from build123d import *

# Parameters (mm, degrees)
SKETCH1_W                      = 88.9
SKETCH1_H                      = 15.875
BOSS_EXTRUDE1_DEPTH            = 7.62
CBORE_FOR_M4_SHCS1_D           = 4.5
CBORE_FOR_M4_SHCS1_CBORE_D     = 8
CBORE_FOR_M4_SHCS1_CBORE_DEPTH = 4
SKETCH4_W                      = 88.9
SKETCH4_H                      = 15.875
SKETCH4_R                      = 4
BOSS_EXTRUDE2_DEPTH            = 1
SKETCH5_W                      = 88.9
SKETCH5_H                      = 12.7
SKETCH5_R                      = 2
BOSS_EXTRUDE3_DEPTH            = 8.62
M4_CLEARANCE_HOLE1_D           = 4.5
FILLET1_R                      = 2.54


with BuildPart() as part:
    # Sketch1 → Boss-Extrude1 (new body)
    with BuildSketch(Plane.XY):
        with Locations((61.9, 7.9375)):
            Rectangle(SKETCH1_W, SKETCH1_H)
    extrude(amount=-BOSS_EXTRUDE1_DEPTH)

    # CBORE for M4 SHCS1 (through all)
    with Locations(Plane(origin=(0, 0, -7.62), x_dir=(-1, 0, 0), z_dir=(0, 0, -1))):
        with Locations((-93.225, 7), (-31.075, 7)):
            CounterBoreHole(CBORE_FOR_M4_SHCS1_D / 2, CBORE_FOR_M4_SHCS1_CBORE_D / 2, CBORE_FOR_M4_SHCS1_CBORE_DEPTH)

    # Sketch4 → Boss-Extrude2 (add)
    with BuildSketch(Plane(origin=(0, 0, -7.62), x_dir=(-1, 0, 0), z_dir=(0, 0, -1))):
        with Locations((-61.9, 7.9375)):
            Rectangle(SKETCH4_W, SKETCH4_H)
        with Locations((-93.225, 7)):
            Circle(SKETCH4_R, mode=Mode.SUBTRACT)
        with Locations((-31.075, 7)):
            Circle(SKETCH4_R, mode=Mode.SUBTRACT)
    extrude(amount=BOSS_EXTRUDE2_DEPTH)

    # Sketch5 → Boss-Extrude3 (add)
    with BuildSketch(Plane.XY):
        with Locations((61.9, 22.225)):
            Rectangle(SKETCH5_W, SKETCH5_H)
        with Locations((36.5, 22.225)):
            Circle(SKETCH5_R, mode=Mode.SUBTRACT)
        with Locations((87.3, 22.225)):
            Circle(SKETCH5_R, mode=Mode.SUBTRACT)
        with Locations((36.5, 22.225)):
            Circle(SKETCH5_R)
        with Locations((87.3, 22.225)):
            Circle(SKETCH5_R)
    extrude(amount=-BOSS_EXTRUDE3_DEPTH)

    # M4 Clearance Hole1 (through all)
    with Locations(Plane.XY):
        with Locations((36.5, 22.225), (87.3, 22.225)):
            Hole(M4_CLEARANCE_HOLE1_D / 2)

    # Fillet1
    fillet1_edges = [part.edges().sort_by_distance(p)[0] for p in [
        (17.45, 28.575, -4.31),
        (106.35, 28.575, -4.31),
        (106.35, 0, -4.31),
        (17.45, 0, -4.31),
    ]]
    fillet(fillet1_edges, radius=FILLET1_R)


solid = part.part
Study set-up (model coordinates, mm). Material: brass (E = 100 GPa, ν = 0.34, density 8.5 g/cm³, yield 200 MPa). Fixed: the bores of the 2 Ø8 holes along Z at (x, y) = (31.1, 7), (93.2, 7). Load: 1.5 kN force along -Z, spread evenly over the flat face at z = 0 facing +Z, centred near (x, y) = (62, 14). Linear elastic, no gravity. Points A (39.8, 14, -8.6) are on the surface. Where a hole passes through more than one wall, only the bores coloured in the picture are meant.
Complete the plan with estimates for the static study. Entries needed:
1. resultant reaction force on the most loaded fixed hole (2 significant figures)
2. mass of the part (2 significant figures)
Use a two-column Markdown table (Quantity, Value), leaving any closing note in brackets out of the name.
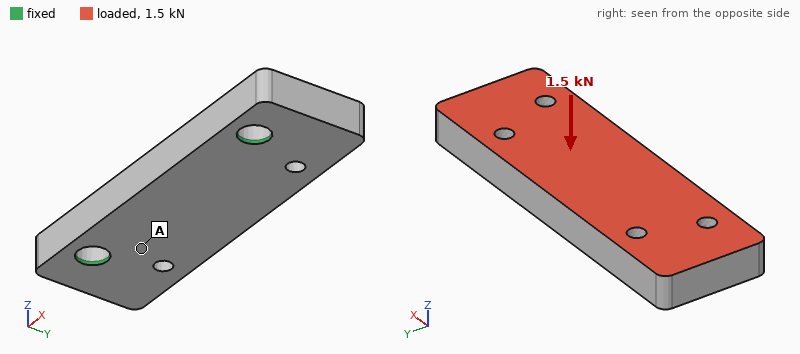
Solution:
| Quantity | Value |
|---|---|
| resultant reaction force on the most loaded fixed hole | 850 N |
| mass of the part | 180 g |
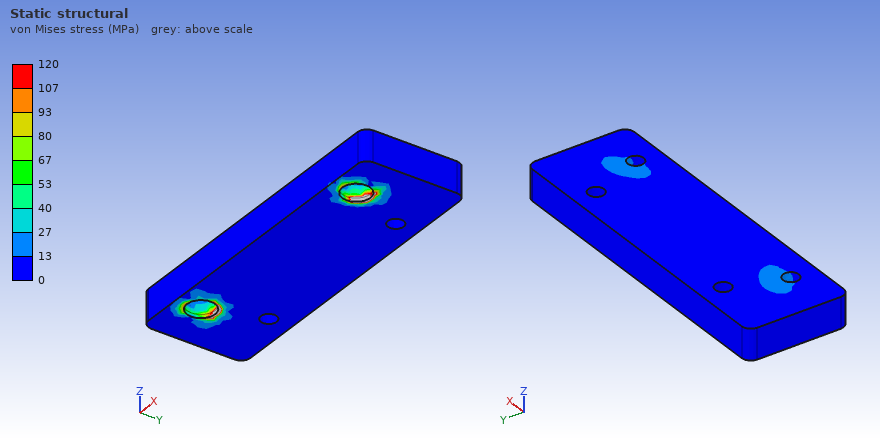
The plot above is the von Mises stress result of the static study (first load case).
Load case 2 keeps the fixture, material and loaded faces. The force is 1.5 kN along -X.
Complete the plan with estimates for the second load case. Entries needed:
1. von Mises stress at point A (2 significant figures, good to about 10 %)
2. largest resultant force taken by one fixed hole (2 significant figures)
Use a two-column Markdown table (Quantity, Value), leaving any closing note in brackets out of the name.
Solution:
| Quantity | Value |
|---|---|
| von Mises stress at point A | 7.8 MPa |
| largest resultant force taken by one fixed hole | 780 N |
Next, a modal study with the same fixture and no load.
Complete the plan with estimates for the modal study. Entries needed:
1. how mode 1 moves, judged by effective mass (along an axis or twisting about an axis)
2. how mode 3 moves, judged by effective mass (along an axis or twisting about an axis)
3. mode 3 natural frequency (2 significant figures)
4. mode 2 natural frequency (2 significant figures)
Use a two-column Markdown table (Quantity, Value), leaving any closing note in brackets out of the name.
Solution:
| Quantity | Value |
|---|---|
| how mode 1 moves, judged by effective mass | along Z |
| how mode 3 moves, judged by effective mass | twisting about Y |
| mode 3 natural frequency | 6200 Hz |
| mode 2 natural frequency | 5900 Hz |
